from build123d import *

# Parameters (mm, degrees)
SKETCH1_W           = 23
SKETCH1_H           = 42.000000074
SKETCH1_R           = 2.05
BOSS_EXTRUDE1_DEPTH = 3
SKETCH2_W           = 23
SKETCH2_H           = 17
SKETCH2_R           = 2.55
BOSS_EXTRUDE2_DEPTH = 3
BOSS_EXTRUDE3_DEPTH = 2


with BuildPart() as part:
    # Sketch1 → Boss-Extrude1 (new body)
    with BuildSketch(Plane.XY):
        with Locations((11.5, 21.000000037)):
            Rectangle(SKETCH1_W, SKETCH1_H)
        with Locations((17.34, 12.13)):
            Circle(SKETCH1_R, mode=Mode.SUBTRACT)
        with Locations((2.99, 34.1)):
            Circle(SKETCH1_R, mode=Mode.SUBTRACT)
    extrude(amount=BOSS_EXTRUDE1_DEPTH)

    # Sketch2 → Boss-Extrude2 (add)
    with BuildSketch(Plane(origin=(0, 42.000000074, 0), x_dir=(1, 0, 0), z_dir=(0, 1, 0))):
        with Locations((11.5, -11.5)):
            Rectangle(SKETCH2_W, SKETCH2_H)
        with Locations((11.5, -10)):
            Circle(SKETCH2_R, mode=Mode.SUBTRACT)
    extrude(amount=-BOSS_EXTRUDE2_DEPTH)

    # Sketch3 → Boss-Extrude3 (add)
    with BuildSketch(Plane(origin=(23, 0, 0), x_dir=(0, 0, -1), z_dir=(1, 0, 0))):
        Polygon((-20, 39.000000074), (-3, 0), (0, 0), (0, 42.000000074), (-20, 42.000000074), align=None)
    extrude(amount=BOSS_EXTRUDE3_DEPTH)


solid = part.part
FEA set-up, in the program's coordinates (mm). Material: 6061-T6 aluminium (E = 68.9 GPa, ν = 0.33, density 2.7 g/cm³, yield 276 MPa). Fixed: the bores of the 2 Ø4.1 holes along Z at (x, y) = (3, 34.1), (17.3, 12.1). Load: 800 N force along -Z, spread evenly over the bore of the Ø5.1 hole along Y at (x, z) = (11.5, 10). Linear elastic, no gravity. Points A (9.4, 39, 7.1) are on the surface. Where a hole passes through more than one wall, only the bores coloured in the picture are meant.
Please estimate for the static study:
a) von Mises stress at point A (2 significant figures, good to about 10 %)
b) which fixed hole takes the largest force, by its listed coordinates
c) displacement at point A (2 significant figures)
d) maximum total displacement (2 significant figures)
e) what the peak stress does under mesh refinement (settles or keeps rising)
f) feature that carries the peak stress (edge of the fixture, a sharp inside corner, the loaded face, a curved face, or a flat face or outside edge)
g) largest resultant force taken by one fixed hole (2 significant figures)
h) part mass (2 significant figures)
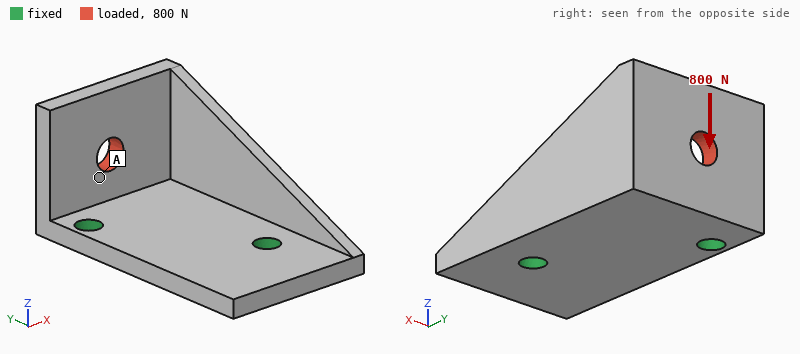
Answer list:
26 MPa
(3, 34.1)
0.064 mm
0.21 mm
keeps rising
edge of the fixture
750 N
13 g
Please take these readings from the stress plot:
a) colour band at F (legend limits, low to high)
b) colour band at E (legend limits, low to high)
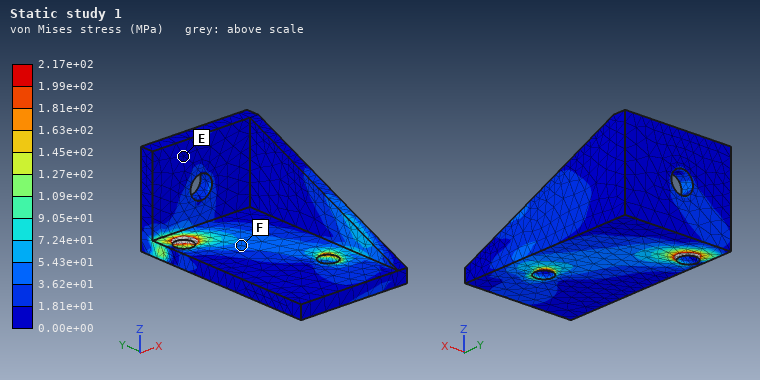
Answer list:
3.62e+01 to 5.43e+01 MPa
0.00e+00 to 1.81e+01 MPa
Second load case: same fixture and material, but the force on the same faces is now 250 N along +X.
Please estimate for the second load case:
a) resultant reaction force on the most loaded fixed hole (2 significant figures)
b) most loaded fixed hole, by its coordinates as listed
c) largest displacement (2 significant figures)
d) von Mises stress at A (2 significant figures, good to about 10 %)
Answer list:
270 N
(3, 34.1)
65 µm
13 MPa
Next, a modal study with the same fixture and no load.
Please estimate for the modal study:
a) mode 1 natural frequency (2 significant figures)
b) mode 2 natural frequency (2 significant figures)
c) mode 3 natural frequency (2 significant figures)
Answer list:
3900 Hz
7600 Hz
9200 Hz
